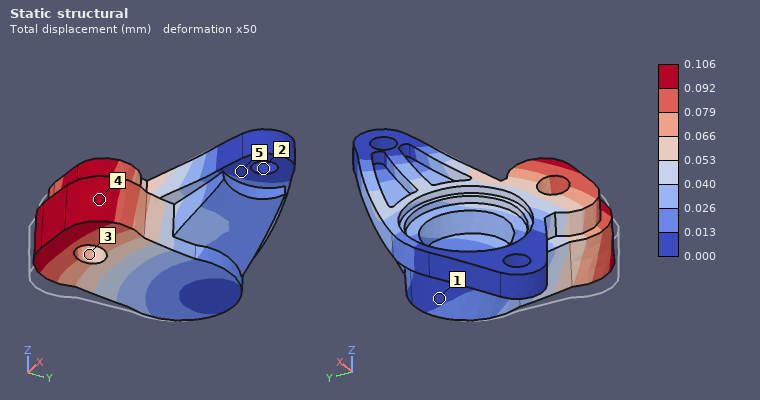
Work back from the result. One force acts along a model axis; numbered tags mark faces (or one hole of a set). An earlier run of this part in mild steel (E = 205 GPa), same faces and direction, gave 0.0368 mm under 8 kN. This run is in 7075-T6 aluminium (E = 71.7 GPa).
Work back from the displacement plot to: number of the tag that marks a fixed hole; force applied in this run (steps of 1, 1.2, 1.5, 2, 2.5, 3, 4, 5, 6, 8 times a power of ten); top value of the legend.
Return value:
2
8 kN
0.106 mm
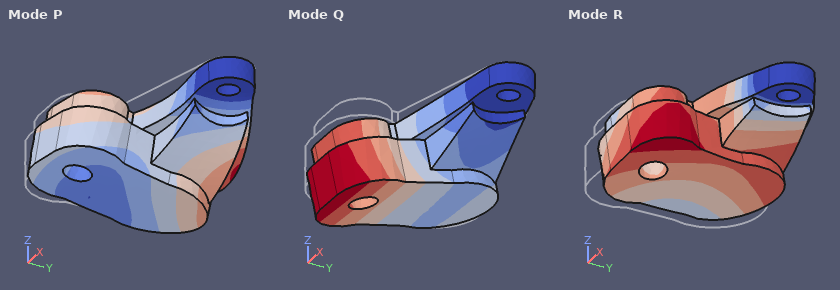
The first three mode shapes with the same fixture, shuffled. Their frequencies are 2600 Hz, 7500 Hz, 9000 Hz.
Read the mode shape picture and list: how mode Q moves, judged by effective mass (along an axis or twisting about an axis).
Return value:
along Z
